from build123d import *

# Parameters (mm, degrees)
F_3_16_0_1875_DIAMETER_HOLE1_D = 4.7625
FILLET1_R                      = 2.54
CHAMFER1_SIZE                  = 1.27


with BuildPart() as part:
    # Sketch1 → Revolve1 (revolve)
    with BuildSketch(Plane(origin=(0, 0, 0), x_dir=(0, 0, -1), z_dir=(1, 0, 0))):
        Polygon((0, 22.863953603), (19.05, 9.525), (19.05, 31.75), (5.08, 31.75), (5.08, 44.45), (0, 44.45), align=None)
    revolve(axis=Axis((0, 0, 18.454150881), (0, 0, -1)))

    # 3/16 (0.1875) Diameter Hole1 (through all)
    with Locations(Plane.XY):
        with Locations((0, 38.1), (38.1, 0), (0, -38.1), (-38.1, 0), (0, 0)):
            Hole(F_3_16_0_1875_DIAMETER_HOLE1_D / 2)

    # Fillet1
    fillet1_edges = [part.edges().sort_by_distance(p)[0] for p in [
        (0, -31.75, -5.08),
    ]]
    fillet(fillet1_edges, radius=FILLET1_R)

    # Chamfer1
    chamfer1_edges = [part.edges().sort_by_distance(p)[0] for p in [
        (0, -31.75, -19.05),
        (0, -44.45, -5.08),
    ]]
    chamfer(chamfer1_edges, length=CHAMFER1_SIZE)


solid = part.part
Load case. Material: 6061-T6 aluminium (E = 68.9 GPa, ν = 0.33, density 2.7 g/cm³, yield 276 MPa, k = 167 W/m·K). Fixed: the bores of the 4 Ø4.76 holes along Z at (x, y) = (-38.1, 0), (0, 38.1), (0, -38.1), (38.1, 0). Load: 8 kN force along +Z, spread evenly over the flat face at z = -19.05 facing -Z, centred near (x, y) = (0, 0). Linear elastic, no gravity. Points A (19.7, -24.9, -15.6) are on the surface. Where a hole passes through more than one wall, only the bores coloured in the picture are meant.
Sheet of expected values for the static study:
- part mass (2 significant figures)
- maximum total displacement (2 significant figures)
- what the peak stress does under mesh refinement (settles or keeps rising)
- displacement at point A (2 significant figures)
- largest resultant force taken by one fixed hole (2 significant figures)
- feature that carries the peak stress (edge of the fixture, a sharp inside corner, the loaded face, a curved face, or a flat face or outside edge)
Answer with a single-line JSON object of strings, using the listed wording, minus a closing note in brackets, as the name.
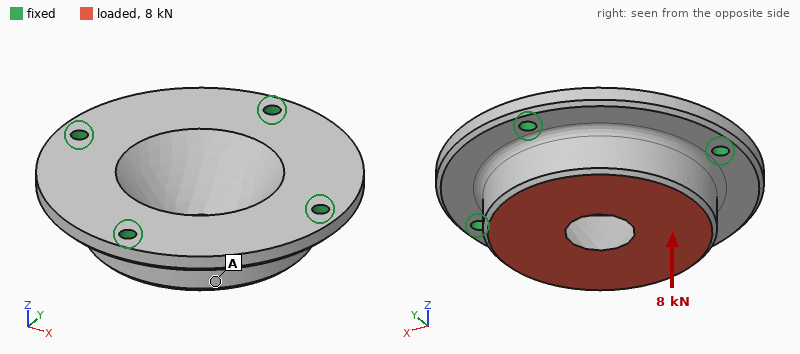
{"part mass": "160 g", "maximum total displacement": "23 µm", "what the peak stress does under mesh refinement": "keeps rising", "displacement at point A": "16 µm", "largest resultant force taken by one fixed hole": "2.5 kN", "feature that carries the peak stress": "edge of the fixture"}
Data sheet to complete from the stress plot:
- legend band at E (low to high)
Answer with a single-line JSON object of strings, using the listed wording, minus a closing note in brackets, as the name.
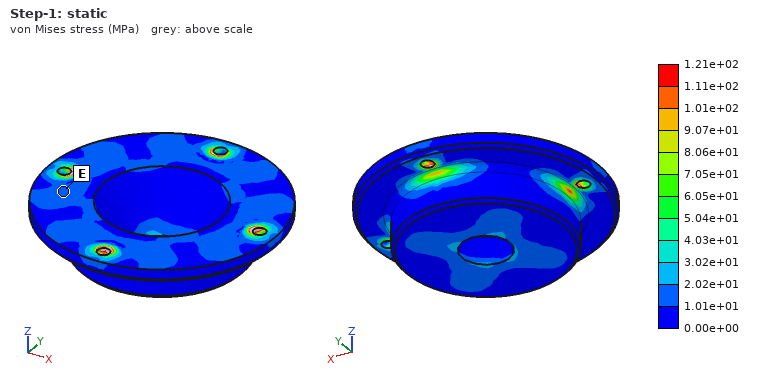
{"legend band at E": "1.01e+01 to 2.02e+01 MPa"}
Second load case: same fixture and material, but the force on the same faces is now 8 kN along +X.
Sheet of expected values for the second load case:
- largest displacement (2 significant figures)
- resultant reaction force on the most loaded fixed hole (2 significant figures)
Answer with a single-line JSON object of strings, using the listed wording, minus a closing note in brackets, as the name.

{"largest displacement": "16 µm", "resultant reaction force on the most loaded fixed hole": "3.0 kN"}
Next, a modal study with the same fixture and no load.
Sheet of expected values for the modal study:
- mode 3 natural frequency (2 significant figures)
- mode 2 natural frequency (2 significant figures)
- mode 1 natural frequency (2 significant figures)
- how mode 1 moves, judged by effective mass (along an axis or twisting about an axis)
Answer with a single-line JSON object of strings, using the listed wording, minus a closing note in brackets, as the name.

{"mode 3 natural frequency": "10 kHz", "mode 2 natural frequency": "10 kHz", "mode 1 natural frequency": "9300 Hz", "how mode 1 moves, judged by effective mass": "along Z"}
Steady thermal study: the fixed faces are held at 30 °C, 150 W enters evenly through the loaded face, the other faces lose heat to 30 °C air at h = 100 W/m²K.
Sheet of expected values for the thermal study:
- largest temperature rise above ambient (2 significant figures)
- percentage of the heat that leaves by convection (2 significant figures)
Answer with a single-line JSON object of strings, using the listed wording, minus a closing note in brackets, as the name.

{"largest temperature rise above ambient": "24 K", "percentage of the heat that leaves by convection": "13 %"}
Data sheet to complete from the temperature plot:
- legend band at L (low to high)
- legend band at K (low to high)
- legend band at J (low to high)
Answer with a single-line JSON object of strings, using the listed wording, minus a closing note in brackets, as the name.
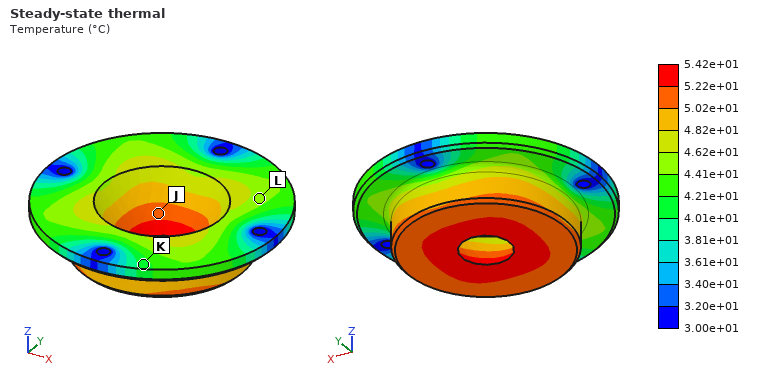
{"legend band at L": "4.41e+01 to 4.62e+01 °C", "legend band at K": "4.01e+01 to 4.21e+01 °C", "legend band at J": "5.02e+01 to 5.22e+01 °C"}
